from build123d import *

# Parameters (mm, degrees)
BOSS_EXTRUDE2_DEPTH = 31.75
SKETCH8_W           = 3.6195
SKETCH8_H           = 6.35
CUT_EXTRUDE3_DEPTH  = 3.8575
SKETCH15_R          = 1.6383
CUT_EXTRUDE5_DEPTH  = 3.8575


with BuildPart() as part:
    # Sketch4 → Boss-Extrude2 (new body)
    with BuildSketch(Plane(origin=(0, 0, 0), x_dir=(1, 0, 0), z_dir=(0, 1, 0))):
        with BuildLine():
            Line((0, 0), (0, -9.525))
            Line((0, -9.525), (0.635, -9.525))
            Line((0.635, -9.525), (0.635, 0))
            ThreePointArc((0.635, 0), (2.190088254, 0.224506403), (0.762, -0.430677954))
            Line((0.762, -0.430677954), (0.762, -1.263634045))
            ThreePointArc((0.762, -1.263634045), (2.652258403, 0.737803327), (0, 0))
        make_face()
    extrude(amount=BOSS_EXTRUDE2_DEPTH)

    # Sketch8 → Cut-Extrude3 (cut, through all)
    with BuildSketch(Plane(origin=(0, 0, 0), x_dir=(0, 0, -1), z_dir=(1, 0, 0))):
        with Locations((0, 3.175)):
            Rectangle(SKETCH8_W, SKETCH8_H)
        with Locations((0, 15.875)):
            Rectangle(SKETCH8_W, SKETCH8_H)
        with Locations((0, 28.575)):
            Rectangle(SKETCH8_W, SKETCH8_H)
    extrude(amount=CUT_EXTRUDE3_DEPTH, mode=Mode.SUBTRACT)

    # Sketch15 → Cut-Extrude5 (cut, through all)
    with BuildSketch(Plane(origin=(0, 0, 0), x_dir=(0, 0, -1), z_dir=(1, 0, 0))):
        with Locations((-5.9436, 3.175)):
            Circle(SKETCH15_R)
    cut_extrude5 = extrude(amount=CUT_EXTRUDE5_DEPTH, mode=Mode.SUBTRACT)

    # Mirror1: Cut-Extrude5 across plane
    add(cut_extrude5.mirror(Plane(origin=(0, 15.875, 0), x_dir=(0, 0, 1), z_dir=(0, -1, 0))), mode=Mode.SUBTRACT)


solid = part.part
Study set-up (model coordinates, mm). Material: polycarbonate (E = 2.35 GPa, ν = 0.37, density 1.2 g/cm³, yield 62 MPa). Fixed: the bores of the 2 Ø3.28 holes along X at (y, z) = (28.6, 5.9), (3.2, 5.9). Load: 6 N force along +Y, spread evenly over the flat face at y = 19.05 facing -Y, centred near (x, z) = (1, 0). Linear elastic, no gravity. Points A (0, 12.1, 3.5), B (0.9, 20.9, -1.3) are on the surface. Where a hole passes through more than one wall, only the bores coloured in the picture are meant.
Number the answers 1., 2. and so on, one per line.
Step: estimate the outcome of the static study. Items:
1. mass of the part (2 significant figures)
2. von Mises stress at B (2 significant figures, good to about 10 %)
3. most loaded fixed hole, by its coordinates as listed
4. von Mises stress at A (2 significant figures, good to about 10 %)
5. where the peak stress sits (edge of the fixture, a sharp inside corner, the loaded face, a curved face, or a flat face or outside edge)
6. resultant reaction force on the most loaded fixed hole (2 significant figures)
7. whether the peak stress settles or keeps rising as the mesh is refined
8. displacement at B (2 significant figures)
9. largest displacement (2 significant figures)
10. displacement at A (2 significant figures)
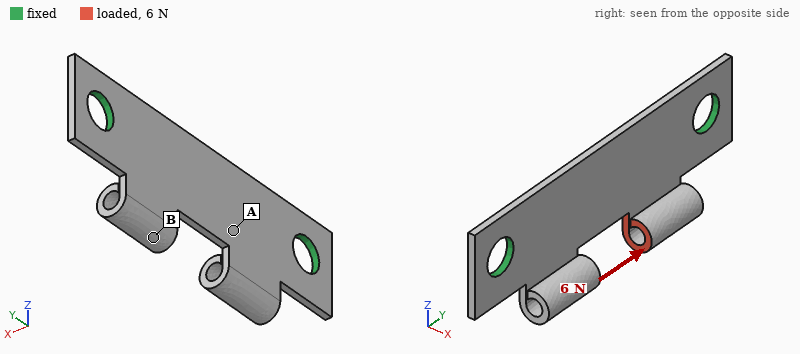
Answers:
1. 0.25 g
2. 6.7 MPa
3. (28.6, 5.9)
4. 2.3 MPa
5. a sharp inside corner
6. 4.5 N
7. keeps rising
8. 0.22 mm
9. 0.36 mm
10. 0.100 mm
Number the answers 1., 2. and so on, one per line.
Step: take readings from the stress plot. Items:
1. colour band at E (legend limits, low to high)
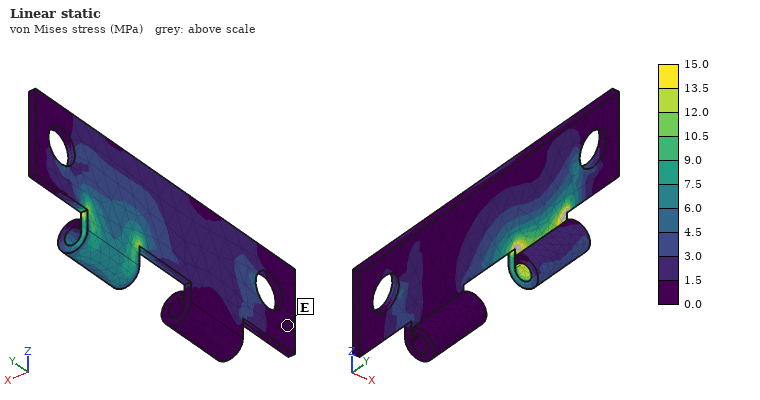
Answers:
1. 0.0 to 1.5 MPa
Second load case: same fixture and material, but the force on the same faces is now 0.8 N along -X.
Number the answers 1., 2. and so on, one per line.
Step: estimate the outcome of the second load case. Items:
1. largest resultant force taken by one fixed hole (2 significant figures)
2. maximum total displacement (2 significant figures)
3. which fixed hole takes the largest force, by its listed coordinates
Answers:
1. 0.57 N
2. 0.40 mm
3. (28.6, 5.9)
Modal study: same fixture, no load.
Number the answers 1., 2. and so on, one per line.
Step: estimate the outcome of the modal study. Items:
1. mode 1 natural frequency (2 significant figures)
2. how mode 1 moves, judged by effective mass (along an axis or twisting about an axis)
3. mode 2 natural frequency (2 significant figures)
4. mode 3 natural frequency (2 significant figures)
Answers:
1. 1200 Hz
2. along X
3. 2000 Hz
4. 2100 Hz
